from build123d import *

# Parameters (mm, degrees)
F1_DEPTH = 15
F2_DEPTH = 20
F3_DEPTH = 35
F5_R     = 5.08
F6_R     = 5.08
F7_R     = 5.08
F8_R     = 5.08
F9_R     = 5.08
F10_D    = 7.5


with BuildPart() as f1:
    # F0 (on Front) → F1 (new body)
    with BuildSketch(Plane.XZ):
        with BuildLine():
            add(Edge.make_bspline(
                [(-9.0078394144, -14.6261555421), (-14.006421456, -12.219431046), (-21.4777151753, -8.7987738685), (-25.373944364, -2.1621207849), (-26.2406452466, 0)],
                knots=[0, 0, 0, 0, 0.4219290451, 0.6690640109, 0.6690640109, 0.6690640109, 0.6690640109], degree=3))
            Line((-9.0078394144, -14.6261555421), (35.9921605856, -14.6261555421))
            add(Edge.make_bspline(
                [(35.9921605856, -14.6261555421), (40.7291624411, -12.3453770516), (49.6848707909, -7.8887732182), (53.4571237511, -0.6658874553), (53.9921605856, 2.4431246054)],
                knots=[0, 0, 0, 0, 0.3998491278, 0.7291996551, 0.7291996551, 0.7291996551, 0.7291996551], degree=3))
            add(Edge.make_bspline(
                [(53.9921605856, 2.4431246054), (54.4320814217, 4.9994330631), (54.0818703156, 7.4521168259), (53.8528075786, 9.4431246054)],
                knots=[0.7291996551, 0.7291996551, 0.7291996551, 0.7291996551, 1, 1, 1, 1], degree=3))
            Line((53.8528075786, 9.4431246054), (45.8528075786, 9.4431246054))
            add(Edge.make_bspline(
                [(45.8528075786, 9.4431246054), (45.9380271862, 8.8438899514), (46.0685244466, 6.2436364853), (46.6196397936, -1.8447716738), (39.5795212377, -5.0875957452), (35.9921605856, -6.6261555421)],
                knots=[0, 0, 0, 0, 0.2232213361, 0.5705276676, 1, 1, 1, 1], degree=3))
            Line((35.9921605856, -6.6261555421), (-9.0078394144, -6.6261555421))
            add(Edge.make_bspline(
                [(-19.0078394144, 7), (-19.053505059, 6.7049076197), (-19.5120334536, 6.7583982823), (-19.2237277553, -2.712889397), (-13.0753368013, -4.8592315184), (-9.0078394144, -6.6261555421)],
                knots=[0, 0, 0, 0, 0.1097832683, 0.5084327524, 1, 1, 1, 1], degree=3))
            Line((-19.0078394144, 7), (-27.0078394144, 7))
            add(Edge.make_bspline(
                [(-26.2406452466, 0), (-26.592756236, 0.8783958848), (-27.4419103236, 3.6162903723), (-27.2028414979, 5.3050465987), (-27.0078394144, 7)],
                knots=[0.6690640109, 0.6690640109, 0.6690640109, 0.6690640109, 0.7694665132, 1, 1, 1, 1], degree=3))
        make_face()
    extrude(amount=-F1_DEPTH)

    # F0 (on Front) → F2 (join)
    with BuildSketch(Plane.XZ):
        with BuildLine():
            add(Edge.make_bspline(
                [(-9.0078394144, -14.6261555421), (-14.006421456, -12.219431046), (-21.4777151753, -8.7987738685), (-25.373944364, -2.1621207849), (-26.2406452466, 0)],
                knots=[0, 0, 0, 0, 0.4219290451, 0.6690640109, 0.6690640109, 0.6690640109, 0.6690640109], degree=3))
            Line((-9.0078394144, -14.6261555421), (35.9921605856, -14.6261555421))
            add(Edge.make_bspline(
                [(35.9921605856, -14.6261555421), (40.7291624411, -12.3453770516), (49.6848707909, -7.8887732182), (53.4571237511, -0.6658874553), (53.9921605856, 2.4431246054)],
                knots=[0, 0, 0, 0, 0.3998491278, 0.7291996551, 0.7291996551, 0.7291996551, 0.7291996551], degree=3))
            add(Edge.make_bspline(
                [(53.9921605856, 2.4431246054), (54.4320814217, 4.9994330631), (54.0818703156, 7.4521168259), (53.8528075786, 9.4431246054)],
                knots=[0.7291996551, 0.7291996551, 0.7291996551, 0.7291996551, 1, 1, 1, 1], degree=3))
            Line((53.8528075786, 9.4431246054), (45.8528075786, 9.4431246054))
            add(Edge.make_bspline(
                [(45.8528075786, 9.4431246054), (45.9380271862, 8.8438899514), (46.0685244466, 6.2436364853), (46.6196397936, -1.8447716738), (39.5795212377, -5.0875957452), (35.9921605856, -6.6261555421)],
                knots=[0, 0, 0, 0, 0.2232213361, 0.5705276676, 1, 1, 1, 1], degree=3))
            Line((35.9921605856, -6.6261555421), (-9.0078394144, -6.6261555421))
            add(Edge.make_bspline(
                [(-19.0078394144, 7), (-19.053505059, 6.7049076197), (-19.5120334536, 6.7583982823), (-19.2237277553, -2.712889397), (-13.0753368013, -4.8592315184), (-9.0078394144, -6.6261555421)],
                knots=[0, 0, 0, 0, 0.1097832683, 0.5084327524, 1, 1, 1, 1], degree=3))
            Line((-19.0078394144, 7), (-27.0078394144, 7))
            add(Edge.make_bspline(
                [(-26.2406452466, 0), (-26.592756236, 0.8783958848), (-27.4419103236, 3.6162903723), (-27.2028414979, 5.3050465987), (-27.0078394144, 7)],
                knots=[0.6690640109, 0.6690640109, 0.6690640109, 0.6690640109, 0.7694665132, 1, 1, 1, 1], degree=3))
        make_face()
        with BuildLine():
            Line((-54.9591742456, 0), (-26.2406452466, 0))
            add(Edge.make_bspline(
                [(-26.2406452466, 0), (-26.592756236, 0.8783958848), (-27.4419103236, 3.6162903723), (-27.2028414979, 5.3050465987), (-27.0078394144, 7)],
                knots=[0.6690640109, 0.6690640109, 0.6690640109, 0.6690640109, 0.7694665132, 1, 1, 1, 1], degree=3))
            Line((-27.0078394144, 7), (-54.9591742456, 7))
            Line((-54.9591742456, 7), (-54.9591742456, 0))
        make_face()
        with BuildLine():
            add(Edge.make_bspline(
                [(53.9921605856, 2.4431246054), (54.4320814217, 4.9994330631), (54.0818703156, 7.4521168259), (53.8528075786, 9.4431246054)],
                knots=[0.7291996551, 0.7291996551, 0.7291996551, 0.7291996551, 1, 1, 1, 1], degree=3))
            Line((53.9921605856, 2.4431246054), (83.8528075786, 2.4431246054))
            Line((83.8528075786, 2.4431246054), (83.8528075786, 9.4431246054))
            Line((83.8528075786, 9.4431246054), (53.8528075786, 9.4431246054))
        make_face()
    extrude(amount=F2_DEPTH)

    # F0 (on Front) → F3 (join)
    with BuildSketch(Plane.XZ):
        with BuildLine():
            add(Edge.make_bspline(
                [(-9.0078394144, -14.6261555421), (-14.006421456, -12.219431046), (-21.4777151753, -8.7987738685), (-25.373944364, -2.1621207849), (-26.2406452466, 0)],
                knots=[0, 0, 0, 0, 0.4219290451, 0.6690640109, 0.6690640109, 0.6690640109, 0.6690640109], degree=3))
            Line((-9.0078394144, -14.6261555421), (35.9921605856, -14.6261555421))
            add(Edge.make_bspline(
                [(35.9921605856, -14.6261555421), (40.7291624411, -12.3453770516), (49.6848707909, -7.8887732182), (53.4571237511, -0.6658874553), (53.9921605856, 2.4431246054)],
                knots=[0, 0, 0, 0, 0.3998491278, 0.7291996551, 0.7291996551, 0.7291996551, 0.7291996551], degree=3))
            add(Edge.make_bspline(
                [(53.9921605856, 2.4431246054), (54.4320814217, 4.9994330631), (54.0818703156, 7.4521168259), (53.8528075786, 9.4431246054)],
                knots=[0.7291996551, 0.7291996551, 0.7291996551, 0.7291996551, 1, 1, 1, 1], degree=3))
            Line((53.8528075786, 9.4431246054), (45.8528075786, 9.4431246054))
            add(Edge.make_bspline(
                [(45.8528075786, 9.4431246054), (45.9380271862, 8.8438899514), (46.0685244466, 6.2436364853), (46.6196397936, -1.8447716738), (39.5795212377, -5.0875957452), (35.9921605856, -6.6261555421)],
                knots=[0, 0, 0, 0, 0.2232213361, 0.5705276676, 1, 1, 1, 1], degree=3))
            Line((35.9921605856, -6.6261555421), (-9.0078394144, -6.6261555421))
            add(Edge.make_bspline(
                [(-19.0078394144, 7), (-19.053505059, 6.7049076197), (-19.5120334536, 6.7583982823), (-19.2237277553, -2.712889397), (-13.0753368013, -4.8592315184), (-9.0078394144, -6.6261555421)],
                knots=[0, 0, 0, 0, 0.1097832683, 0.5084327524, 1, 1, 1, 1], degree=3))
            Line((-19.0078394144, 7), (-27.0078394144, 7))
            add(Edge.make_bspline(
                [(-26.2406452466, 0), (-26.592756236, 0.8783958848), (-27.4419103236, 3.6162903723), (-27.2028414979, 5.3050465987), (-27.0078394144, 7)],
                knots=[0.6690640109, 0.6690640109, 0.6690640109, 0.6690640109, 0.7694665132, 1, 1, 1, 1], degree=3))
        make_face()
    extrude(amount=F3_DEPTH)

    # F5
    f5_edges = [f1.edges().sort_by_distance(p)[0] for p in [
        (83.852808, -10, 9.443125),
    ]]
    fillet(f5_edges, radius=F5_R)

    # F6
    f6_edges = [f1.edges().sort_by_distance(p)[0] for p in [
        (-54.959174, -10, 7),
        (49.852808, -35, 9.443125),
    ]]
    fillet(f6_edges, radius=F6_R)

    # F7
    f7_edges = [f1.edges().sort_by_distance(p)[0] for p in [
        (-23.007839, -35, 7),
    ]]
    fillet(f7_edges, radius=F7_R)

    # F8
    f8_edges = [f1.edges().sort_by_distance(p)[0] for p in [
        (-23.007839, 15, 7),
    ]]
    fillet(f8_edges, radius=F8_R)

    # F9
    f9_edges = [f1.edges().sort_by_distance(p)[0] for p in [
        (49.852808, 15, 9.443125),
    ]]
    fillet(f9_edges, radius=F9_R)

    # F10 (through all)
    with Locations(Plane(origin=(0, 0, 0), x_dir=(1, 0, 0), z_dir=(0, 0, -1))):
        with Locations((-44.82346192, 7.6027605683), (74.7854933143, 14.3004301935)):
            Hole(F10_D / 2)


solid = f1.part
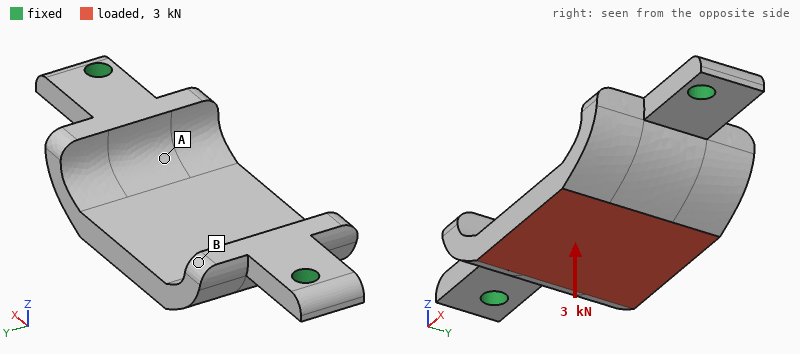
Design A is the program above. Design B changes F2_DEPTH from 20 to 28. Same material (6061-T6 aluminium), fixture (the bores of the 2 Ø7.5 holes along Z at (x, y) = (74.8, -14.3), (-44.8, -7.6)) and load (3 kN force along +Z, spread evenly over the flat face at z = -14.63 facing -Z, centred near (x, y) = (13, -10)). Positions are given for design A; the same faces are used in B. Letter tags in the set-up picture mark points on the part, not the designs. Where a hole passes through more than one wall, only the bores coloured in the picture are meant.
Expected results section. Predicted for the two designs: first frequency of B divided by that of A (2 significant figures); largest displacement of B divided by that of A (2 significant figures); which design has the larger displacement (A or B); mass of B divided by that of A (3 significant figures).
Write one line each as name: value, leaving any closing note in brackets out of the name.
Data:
first frequency of B divided by that of A: 1.2
largest displacement of B divided by that of A: 1.1
which design has the larger displacement: B
mass of B divided by that of A: 1.07
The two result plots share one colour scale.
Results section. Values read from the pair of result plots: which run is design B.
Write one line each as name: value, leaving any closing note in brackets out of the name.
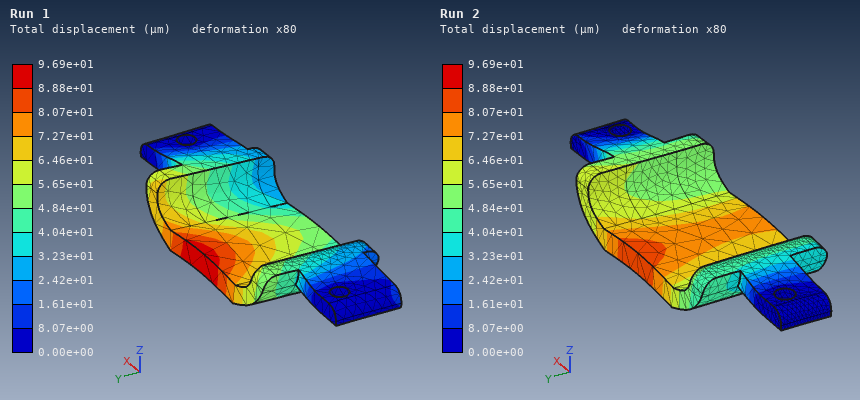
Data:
which run is design B: Run 1
